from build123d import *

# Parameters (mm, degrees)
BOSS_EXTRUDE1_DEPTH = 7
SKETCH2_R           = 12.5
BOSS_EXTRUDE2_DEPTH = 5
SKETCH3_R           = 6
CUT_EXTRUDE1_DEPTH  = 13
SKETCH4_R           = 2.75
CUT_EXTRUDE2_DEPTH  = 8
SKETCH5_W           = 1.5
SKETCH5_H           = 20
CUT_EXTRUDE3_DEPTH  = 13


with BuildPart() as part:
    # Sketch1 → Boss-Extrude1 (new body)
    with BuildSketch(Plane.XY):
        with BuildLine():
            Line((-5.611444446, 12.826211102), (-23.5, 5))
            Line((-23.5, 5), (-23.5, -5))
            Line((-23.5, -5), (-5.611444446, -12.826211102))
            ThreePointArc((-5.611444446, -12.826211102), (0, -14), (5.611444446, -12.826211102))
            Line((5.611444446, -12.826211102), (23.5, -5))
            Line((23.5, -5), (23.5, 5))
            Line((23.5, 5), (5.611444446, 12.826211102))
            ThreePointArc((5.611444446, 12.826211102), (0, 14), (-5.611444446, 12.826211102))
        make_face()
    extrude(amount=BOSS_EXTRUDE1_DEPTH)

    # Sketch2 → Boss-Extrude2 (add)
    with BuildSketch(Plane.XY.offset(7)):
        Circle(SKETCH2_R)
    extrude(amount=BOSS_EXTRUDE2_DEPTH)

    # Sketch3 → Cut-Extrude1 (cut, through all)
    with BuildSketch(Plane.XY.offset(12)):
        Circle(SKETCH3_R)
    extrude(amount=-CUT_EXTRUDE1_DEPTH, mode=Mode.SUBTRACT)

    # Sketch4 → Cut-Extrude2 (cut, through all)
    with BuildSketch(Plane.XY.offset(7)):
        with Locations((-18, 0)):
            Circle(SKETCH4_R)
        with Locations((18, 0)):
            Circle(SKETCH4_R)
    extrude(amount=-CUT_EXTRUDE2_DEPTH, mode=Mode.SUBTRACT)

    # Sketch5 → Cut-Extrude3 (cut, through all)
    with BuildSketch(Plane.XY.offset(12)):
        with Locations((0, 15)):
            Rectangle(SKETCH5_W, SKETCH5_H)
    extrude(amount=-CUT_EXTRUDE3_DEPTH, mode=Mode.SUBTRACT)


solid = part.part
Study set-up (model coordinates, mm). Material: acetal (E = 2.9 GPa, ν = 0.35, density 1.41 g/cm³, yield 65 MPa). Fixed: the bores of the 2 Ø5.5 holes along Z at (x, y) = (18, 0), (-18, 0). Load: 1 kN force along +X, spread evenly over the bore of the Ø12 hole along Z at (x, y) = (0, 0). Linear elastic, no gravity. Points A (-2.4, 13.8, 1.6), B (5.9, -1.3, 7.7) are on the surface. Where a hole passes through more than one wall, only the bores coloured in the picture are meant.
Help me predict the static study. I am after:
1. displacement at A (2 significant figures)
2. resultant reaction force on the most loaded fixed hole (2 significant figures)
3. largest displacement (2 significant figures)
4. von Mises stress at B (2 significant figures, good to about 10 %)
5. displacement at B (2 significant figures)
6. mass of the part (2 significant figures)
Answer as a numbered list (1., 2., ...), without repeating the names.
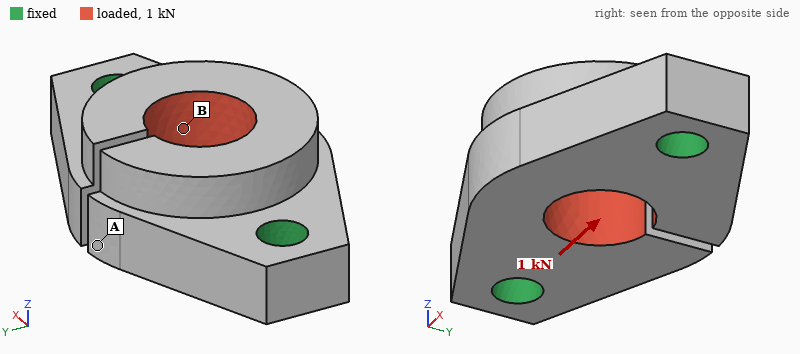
1. 53 µm
2. 500 N
3. 75 µm
4. 5.1 MPa
5. 34 µm
6. 10 g
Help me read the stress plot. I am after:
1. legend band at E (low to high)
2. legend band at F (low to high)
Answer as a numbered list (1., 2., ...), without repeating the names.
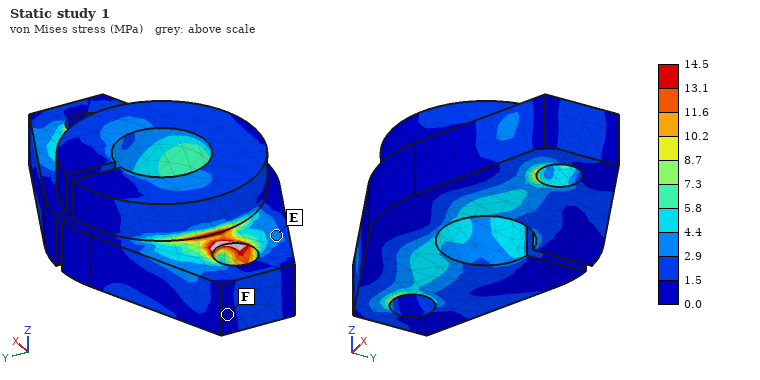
1. 2.9 to 4.4 MPa
2. 0.0 to 1.5 MPa
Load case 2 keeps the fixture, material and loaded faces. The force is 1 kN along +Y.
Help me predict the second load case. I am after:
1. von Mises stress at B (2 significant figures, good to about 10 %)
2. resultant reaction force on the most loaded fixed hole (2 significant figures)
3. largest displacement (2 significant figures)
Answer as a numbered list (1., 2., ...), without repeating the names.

1. 6.7 MPa
2. 630 N
3. 0.21 mm
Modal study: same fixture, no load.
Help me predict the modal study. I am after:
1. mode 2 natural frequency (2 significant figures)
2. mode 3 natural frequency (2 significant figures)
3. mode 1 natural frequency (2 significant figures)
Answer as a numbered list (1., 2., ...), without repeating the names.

1. 4800 Hz
2. 4900 Hz
3. 4500 Hz
